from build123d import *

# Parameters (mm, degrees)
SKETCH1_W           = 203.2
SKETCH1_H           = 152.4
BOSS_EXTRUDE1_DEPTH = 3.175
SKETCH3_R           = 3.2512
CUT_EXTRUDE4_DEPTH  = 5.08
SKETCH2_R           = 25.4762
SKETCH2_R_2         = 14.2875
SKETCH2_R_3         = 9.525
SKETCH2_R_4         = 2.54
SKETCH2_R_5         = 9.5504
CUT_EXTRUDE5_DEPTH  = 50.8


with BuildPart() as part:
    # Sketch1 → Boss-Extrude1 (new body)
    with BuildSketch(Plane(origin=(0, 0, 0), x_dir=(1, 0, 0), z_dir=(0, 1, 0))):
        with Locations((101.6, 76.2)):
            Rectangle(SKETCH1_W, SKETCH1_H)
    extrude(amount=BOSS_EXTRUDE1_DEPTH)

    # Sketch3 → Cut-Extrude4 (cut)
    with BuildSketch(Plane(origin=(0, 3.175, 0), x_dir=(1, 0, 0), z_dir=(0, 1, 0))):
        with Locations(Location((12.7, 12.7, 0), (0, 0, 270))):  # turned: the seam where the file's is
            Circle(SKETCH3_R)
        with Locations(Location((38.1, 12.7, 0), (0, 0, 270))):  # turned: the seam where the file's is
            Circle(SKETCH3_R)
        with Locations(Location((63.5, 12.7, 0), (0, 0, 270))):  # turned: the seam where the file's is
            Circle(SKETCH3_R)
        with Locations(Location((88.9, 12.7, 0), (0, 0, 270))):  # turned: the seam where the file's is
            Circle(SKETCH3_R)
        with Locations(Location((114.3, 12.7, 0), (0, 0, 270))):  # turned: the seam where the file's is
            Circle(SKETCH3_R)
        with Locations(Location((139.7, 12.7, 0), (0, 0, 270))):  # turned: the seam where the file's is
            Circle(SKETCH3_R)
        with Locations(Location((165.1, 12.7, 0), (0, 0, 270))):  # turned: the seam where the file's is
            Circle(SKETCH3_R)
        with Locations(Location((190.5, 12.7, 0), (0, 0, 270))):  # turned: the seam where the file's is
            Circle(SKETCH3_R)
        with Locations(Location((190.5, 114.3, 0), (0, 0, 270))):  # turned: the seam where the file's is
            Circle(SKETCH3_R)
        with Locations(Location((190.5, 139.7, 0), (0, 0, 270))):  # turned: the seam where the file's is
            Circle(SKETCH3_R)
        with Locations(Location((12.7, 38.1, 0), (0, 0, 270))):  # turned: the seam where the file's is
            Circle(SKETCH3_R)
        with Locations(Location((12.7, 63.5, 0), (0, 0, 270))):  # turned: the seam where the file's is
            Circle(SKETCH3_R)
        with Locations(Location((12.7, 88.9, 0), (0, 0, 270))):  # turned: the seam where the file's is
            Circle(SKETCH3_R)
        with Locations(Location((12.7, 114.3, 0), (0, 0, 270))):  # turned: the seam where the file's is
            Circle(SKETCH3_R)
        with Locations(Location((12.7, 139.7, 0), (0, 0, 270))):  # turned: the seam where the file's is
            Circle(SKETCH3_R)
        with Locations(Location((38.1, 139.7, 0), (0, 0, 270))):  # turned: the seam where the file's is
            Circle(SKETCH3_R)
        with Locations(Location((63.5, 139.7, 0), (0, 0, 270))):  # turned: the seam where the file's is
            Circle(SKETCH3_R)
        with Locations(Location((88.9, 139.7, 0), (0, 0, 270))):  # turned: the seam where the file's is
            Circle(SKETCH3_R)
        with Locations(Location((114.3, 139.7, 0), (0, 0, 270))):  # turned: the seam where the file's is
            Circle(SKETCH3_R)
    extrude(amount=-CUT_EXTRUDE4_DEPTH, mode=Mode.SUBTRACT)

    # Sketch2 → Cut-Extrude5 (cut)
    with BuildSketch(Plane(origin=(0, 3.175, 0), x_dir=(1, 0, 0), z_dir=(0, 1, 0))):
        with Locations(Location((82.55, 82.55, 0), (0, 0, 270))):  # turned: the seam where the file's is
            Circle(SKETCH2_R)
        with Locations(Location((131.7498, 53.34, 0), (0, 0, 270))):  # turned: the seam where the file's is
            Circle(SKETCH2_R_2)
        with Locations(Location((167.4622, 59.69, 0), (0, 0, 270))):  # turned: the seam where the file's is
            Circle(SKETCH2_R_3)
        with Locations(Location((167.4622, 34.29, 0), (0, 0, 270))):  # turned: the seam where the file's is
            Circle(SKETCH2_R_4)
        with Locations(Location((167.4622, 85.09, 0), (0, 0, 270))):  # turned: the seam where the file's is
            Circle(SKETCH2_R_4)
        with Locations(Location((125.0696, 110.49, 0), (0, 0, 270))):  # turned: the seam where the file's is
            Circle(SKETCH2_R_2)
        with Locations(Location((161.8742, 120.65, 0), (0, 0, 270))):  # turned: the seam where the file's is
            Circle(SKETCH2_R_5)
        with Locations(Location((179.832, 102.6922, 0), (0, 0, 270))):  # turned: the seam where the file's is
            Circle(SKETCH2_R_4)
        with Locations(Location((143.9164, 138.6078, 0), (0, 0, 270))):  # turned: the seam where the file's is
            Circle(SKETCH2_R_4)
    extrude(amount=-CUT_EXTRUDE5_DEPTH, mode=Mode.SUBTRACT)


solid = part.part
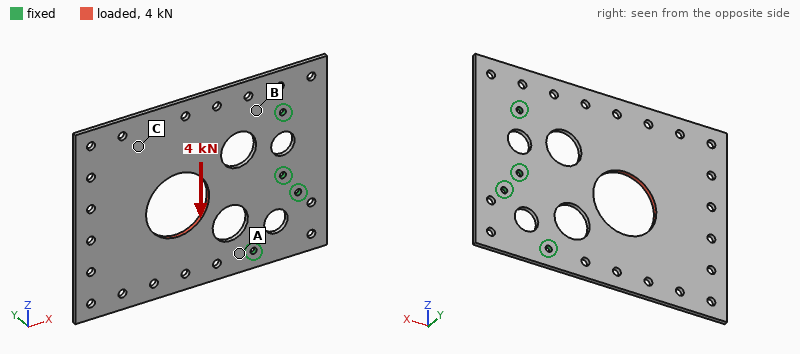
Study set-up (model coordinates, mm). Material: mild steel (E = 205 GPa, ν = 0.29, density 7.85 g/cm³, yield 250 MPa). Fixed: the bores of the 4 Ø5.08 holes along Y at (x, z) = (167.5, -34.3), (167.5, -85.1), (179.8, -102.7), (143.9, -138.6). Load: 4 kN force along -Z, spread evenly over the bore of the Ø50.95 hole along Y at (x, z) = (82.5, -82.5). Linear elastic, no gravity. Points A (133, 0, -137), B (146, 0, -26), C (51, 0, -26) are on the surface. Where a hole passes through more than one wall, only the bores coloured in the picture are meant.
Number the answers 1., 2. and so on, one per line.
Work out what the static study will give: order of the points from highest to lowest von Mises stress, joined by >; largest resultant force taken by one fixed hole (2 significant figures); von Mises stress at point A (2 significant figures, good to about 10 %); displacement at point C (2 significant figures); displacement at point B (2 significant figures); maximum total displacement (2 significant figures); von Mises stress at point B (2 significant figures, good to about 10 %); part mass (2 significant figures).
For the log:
1. A > B > C
2. 3.2 kN
3. 40 MPa
4. 35 µm
5. 8.6 µm
6. 43 µm
7. 23 MPa
8. 660 g
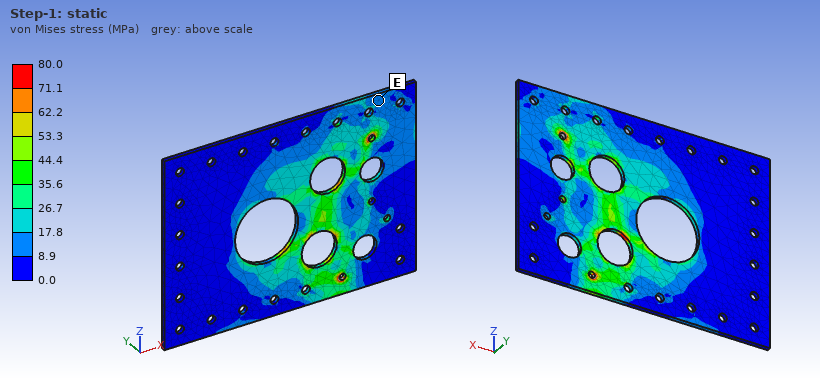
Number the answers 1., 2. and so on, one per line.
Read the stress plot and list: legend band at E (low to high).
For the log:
1. 8.9 to 17.8 MPa
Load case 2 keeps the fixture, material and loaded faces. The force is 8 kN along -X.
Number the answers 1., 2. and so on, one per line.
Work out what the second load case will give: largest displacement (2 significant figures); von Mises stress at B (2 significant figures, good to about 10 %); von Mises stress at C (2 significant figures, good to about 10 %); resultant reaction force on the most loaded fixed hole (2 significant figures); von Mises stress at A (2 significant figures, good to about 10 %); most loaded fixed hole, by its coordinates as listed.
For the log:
1. 19 µm
2. 30 MPa
3. 7.4 MPa
4. 3.3 kN
5. 42 MPa
6. (167.5, -34.3)
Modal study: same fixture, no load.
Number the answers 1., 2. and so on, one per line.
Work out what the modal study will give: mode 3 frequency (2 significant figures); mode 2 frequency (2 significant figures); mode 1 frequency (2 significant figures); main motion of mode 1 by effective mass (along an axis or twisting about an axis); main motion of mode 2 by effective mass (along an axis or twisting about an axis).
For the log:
1. 600 Hz
2. 240 Hz
3. 90 Hz
4. along Y
5. twisting about X
